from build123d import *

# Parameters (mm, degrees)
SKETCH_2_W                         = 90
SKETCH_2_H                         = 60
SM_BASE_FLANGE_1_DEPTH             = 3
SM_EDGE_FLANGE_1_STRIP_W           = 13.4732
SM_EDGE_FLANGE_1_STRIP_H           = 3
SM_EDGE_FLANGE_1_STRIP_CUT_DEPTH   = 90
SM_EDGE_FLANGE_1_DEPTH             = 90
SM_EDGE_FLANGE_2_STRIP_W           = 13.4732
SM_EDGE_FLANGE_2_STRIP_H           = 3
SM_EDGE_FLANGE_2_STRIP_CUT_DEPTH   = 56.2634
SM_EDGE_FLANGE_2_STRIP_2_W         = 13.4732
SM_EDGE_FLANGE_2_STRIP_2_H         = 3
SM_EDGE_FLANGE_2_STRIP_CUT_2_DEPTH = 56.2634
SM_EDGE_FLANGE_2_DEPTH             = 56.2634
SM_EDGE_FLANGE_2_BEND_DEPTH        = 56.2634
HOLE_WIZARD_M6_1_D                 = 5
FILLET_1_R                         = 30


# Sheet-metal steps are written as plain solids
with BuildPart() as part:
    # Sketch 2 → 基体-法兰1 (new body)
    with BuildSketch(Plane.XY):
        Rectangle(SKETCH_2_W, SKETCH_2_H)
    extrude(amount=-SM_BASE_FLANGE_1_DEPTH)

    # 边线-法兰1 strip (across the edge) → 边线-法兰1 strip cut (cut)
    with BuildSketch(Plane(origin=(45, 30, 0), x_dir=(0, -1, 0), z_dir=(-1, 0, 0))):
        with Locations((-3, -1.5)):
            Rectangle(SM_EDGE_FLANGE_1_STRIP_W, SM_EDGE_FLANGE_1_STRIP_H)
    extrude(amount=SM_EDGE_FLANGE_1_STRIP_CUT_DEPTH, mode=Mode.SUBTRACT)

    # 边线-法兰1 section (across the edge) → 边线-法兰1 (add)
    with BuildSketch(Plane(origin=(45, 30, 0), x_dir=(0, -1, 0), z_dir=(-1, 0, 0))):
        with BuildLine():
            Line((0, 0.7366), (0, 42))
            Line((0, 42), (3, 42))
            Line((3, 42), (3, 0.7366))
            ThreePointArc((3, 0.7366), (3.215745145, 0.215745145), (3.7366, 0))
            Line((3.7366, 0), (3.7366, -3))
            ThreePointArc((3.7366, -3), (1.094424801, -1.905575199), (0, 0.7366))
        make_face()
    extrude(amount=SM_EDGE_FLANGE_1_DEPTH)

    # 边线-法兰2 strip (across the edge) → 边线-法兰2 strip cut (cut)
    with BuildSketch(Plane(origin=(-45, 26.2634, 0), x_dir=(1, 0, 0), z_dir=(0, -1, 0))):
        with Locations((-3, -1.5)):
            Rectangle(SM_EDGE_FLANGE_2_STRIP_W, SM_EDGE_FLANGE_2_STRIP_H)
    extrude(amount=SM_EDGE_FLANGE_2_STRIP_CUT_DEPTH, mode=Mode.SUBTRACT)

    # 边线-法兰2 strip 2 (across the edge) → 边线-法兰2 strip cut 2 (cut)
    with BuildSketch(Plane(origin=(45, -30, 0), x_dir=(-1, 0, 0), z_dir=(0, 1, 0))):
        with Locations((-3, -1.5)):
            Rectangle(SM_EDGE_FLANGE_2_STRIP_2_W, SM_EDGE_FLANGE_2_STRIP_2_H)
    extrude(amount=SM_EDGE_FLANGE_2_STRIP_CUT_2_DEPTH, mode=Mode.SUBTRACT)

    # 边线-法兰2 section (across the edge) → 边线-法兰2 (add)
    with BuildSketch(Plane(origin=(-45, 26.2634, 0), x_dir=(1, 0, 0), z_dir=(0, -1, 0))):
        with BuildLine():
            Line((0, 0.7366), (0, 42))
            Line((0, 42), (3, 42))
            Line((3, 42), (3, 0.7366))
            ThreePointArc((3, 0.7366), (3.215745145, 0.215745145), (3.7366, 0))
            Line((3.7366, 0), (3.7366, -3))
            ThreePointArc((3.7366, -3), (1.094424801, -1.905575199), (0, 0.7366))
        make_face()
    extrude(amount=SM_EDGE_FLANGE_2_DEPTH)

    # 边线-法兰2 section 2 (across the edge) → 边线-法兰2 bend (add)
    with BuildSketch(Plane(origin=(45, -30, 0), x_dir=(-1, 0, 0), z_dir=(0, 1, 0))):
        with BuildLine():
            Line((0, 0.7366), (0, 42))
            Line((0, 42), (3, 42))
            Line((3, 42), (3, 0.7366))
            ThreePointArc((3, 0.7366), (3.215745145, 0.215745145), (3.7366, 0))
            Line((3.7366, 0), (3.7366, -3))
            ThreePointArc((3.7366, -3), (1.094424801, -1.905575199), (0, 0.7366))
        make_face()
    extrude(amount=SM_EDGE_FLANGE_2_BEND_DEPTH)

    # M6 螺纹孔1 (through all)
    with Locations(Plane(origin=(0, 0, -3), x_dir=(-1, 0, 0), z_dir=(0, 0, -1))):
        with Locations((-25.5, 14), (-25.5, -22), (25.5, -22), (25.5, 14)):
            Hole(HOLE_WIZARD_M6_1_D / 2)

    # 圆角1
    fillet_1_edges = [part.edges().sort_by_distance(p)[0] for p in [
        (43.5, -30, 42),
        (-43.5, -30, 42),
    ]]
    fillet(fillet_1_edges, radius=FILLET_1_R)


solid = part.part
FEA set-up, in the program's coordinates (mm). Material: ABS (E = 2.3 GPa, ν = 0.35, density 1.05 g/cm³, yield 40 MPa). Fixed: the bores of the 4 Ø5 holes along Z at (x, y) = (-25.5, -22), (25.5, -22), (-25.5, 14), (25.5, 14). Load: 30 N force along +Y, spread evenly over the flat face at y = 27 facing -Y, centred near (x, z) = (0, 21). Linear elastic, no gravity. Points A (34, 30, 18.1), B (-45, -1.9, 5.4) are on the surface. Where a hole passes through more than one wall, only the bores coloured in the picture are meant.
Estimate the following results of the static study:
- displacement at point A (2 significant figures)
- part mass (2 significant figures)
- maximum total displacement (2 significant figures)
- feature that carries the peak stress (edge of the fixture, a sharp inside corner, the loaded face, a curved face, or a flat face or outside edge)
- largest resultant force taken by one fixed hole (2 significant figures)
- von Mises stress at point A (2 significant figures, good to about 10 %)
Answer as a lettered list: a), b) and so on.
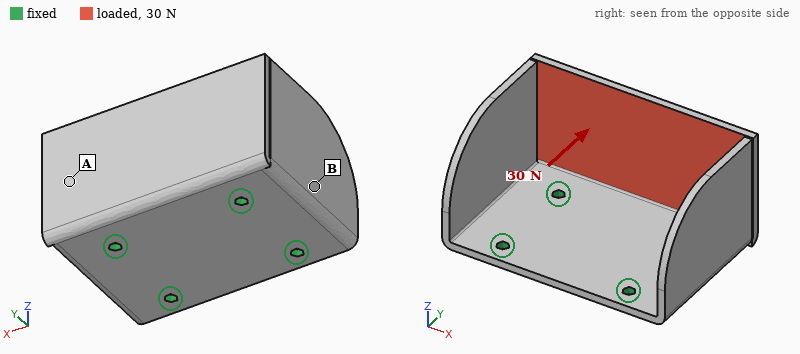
a) 0.50 mm
b) 42 g
c) 1.3 mm
d) a curved face
e) 13 N
f) 1.5 MPa
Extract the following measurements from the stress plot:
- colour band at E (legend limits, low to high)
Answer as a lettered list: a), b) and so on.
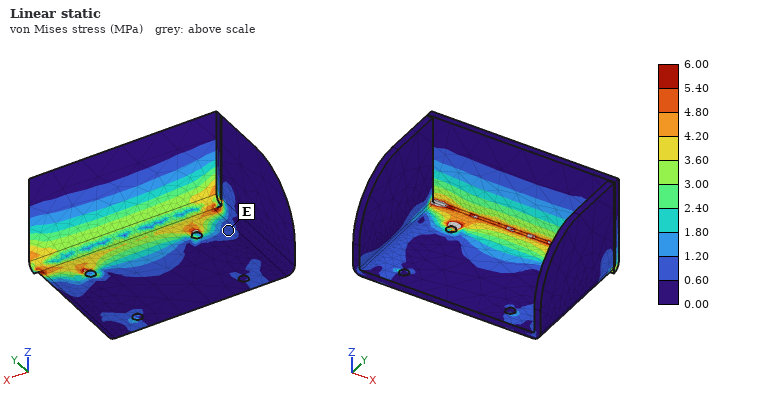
a) 0.60 to 1.20 MPa
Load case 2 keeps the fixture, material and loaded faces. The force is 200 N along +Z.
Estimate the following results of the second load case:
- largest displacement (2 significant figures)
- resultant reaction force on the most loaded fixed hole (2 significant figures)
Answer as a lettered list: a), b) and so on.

a) 0.92 mm
b) 120 N
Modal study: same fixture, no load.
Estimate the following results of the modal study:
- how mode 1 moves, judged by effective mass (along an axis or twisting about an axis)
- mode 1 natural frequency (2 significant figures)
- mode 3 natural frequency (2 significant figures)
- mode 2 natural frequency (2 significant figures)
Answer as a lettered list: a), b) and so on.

a) along Y
b) 270 Hz
c) 300 Hz
d) 290 Hz
